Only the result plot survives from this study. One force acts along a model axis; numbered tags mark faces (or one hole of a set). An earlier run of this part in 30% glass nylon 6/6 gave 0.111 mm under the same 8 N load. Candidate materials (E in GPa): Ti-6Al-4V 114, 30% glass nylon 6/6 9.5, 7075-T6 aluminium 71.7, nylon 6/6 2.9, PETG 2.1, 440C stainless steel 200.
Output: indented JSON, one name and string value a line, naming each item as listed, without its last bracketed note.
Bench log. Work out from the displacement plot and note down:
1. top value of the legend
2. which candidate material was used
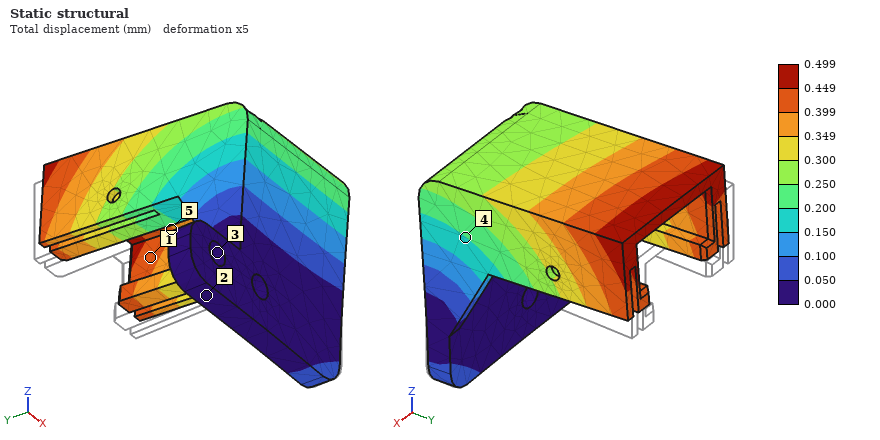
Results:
{
  "top value of the legend": "0.499 mm",
  "which candidate material was used": "PETG"
}
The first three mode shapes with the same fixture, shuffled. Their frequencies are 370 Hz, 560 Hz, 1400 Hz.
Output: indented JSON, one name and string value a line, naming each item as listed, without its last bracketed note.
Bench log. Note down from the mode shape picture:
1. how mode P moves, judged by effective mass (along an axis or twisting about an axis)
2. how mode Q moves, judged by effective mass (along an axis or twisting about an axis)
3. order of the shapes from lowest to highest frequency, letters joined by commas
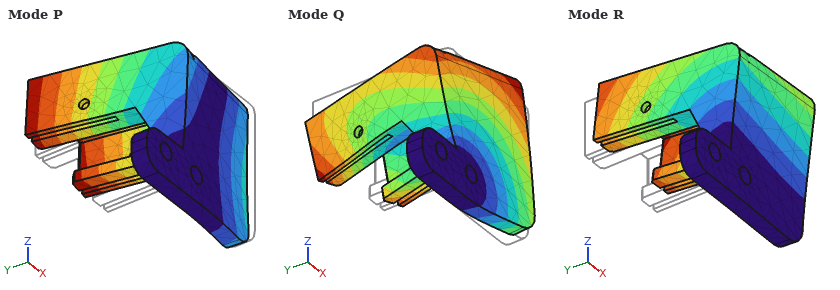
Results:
{
  "how mode P moves, judged by effective mass": "along X",
  "how mode Q moves, judged by effective mass": "along X",
  "order of the shapes from lowest to highest frequency, letters joined by commas": "R, P, Q"
}
